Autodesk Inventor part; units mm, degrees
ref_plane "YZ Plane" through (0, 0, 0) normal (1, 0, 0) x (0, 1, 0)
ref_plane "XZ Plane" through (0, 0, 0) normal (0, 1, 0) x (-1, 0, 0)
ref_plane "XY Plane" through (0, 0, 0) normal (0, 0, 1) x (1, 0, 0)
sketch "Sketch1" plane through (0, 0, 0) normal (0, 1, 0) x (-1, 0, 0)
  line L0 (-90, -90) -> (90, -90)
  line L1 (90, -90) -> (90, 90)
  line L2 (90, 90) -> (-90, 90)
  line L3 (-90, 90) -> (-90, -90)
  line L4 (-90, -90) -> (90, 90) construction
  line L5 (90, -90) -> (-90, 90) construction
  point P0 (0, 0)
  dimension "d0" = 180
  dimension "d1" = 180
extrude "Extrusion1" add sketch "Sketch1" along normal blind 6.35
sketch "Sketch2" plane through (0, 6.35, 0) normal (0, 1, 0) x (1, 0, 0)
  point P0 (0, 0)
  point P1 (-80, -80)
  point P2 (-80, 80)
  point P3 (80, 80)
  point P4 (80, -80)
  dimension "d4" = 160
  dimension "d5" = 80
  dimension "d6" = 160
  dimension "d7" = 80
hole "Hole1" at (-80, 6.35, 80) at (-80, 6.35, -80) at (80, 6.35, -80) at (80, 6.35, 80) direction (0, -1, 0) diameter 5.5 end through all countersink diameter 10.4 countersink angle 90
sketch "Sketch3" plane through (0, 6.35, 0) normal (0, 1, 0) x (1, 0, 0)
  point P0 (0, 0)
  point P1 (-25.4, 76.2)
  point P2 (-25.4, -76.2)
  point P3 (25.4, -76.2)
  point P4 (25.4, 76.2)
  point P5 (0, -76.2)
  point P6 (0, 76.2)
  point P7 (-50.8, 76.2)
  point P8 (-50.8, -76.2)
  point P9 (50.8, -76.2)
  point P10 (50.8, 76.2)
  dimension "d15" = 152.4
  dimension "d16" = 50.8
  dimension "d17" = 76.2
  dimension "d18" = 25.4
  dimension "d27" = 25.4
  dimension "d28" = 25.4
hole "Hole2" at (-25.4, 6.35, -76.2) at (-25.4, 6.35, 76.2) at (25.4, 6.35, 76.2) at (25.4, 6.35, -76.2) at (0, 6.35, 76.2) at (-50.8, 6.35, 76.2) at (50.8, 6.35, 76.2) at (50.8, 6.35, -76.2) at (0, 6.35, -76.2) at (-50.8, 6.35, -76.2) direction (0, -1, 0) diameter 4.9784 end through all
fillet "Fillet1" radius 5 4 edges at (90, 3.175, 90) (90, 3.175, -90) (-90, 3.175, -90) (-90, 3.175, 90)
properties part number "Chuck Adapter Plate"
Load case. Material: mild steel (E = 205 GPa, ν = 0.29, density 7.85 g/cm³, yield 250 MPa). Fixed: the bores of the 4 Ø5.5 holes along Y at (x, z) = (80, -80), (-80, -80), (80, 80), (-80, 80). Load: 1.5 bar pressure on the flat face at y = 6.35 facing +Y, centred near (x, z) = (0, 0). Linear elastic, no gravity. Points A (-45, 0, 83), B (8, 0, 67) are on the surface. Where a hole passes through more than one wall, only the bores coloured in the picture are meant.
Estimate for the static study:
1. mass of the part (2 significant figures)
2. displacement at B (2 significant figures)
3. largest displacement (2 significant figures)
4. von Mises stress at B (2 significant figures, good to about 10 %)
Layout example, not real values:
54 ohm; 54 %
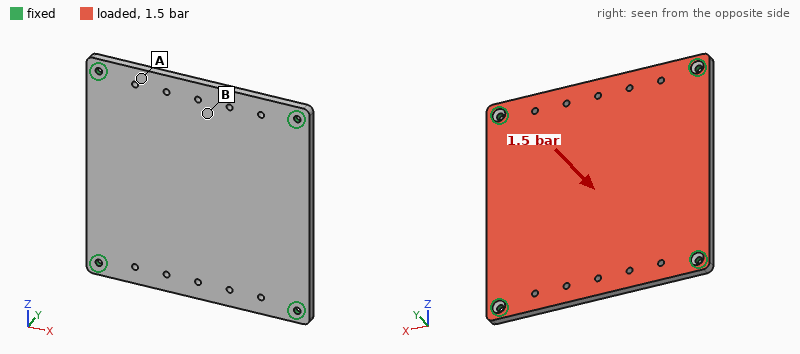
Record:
1.6 kg; 0.14 mm; 0.21 mm; 35 MPa
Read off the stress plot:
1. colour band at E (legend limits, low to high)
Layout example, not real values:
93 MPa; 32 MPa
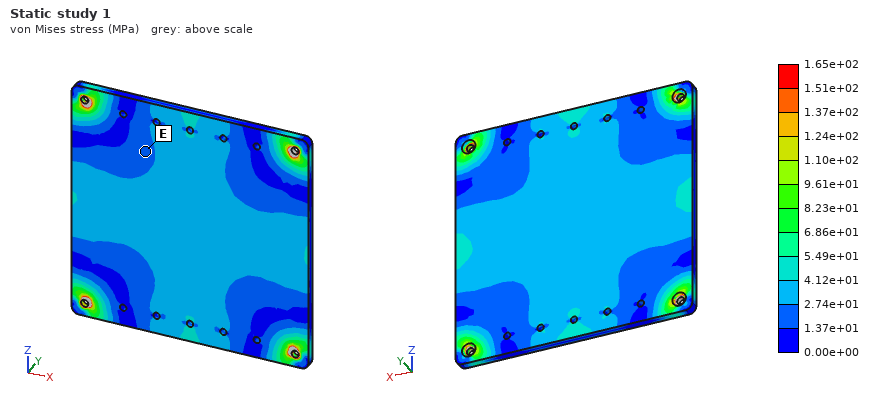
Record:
1.37e+01 to 2.74e+01 MPa
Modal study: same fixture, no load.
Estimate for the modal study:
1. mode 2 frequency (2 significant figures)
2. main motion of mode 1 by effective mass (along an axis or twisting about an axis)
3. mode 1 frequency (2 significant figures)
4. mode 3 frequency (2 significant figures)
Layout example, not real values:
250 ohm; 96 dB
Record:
1300 Hz; along Y; 710 Hz; 1300 Hz
